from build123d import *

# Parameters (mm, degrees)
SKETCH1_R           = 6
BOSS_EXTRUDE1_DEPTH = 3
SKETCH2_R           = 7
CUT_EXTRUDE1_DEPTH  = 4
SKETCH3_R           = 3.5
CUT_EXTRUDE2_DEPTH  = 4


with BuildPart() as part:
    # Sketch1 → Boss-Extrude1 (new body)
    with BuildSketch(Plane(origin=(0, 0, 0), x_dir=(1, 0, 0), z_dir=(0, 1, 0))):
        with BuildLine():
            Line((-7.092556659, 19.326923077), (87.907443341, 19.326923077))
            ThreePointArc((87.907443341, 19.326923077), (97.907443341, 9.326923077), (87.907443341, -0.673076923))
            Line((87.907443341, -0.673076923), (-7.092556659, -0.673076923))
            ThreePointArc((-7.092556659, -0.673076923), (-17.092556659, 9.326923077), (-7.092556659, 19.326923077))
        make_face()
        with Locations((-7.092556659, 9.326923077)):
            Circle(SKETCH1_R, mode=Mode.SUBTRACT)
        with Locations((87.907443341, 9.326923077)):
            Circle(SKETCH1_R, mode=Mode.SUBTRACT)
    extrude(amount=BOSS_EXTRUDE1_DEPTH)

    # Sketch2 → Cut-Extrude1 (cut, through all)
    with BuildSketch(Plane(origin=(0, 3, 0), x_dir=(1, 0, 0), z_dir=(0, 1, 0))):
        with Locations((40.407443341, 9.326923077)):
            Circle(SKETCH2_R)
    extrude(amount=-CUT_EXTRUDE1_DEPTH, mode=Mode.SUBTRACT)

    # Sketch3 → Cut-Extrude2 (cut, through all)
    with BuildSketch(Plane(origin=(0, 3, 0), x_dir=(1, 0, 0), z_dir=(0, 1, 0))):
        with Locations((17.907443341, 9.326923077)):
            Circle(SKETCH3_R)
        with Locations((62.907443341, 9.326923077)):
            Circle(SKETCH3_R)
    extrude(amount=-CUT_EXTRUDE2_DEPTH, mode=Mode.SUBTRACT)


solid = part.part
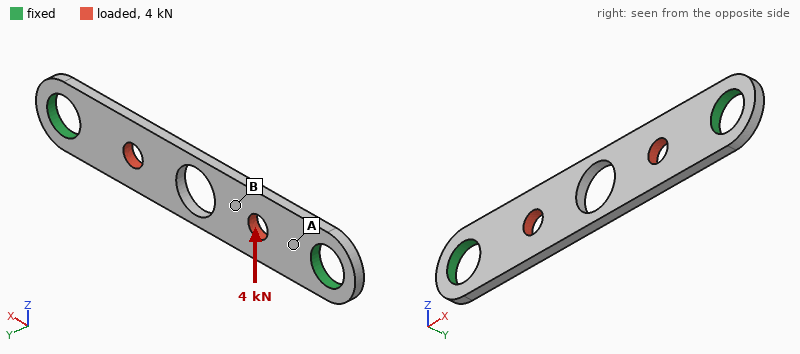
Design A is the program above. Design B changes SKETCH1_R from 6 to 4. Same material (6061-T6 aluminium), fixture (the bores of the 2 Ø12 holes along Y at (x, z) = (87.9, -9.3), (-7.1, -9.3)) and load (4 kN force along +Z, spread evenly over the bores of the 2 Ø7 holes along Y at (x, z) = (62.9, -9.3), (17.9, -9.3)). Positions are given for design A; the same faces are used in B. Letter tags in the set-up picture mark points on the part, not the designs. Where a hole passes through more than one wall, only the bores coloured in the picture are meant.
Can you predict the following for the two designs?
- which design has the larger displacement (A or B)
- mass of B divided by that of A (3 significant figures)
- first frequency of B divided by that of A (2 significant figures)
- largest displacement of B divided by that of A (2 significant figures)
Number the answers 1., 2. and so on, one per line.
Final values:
1. B
2. 1.07
3. 0.90
4. 1.3
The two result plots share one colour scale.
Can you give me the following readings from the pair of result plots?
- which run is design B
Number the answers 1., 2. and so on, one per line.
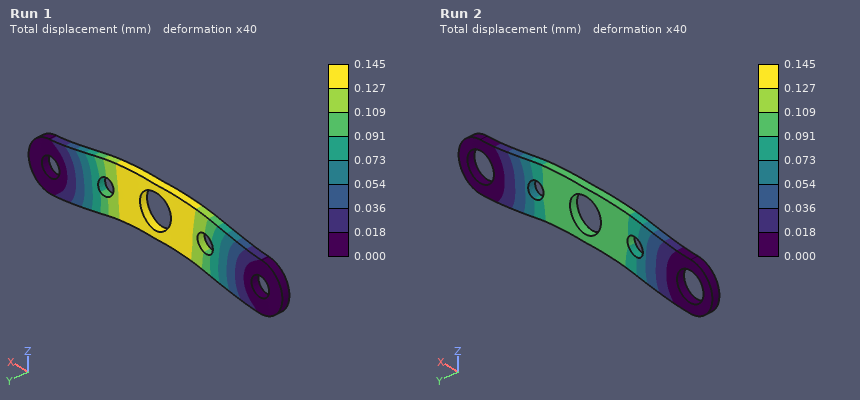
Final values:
1. Run 1
